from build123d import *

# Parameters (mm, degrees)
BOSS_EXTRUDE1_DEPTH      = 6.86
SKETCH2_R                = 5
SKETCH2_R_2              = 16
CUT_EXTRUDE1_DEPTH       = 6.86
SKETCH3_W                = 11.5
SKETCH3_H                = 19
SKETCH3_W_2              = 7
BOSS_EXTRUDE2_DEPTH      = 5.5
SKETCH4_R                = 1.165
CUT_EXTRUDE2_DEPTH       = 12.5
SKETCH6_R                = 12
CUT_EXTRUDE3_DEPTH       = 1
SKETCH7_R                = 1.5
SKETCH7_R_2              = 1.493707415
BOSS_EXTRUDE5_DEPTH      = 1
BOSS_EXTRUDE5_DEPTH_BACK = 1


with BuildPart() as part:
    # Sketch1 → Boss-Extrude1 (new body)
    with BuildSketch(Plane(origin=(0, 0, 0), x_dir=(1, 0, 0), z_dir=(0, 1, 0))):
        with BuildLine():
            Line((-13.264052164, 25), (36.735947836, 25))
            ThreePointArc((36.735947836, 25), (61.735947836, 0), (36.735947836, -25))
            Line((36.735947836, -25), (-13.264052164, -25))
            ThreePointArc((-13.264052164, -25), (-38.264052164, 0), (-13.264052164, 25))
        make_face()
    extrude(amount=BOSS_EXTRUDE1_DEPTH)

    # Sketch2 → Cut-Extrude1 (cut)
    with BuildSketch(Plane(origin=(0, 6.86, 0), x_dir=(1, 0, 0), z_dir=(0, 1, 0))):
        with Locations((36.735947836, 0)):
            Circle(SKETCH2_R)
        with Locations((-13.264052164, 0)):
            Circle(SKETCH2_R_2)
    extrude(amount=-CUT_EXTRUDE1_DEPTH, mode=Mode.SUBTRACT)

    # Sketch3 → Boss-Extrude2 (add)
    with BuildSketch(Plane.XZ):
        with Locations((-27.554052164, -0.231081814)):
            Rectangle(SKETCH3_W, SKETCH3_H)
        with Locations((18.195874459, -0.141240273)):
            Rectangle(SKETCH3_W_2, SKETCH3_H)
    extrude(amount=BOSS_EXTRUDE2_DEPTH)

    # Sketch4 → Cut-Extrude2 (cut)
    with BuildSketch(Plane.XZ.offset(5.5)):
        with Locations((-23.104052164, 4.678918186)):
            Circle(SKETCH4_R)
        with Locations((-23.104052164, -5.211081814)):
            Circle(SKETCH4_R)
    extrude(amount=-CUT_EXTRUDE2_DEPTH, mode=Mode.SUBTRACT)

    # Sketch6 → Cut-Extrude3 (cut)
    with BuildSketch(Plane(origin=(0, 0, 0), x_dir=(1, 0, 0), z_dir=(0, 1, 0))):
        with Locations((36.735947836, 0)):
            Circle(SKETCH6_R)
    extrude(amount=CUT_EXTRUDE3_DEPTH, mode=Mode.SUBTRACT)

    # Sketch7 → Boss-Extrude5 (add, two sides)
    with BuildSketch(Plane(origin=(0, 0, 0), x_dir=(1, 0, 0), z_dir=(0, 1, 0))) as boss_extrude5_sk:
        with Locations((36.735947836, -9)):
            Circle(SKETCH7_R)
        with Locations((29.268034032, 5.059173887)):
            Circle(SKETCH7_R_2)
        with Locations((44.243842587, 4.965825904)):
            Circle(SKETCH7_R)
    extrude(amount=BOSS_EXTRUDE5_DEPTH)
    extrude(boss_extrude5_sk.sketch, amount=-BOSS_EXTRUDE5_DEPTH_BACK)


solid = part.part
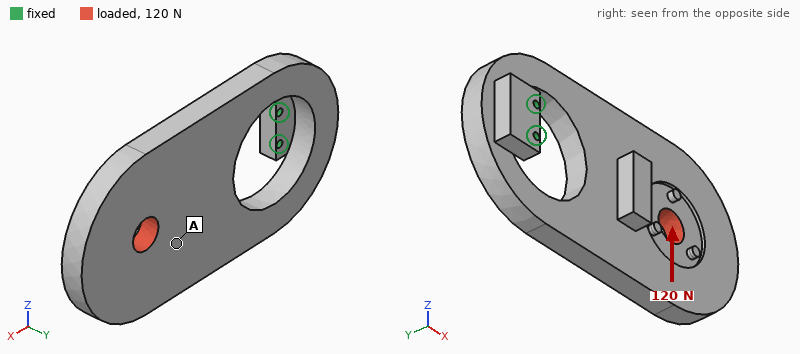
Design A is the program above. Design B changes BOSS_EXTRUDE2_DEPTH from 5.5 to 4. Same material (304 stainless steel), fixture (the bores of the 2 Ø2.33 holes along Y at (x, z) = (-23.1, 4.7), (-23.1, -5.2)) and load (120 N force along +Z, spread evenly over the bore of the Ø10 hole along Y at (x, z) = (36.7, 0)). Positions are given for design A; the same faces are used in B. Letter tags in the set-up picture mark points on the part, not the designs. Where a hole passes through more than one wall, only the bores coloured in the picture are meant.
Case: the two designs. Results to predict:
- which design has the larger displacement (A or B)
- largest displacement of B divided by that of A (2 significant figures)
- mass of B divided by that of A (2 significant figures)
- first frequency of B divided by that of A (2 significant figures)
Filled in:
B
1.1
0.98
0.86
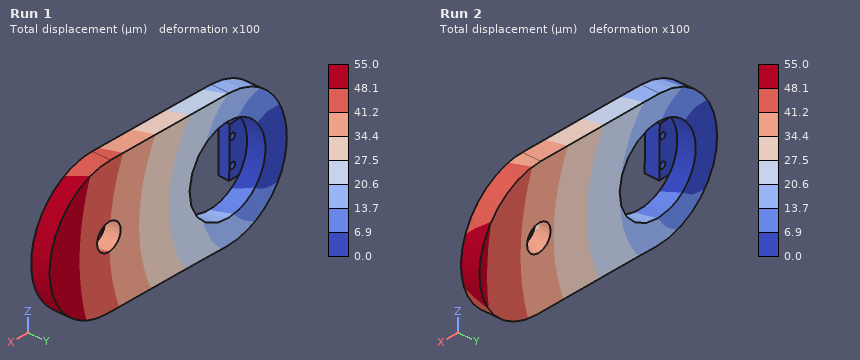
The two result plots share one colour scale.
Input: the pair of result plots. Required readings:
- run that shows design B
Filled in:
Run 1
